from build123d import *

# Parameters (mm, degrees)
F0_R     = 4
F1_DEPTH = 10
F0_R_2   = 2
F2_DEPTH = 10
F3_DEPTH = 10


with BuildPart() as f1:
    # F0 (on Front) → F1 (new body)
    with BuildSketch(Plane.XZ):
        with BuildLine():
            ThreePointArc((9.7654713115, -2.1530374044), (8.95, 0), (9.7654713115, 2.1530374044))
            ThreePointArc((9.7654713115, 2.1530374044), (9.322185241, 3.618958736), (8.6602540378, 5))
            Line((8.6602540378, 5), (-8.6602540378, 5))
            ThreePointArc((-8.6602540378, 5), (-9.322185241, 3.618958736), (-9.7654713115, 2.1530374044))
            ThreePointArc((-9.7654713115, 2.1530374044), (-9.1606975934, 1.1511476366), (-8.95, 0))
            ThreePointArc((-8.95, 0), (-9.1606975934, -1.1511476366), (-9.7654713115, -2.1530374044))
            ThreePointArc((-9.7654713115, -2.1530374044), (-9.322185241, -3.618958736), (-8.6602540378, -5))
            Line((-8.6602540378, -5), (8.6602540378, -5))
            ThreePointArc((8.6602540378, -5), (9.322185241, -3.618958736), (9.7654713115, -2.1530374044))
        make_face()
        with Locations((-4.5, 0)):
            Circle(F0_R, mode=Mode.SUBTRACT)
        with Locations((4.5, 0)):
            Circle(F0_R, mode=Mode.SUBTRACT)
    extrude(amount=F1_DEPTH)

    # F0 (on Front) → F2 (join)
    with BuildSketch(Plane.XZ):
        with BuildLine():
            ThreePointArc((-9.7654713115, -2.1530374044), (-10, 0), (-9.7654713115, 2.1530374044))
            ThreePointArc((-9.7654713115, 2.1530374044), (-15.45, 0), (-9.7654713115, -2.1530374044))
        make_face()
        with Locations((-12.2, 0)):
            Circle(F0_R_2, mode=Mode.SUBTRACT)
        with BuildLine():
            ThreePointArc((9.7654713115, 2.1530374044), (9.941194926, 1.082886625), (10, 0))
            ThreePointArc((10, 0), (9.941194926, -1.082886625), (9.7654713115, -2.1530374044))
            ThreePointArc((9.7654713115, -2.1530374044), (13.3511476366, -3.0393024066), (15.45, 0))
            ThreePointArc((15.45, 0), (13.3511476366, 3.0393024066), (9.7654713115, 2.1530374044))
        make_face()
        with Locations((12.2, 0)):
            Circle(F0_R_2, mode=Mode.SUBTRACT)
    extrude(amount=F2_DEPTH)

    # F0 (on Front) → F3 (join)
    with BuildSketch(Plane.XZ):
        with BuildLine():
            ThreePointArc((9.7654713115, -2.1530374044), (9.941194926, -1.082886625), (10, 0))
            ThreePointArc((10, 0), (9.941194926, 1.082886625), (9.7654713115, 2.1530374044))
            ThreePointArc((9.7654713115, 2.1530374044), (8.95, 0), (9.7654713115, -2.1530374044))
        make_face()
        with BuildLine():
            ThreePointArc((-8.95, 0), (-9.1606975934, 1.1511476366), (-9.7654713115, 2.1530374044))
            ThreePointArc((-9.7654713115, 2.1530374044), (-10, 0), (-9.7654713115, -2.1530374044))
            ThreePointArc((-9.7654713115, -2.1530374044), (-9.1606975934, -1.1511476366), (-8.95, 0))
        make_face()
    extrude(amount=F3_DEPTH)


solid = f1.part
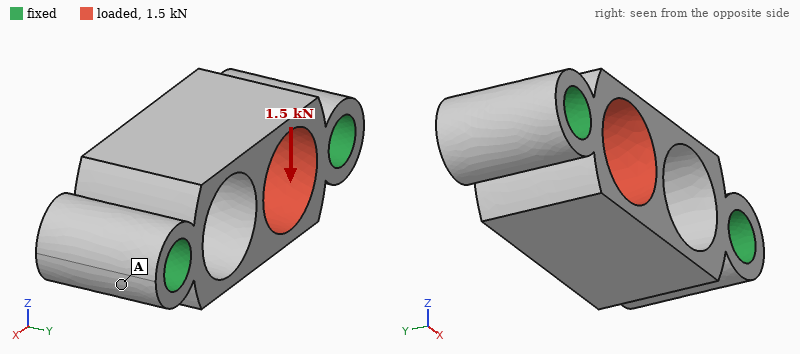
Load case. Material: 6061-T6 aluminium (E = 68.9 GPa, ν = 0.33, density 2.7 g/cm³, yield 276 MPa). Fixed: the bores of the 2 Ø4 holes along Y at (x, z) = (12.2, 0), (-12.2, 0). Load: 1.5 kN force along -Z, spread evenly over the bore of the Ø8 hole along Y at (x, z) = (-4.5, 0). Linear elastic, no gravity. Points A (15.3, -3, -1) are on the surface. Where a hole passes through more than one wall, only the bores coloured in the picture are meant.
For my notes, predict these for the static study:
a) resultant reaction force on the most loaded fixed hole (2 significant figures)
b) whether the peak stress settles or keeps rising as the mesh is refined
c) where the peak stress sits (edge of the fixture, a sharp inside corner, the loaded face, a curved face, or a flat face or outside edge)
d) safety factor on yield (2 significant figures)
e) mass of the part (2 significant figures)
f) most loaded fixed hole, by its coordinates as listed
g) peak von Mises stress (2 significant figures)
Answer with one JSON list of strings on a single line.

["1.1 kN", "settles", "a flat face or outside edge", "1.9", "3.4 g", "(-12.2, 0)", "150 MPa"]
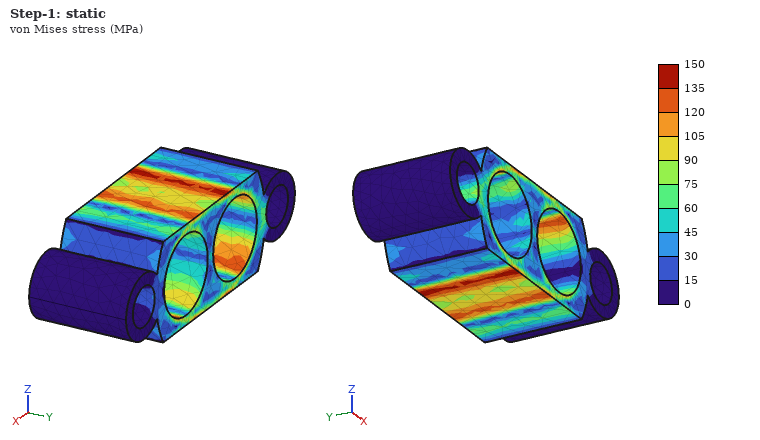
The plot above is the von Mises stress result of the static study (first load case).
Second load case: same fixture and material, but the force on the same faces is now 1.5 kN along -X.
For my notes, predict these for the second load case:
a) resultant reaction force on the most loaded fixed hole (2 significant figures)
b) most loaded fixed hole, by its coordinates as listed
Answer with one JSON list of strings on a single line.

["1.0 kN", "(-12.2, 0)"]
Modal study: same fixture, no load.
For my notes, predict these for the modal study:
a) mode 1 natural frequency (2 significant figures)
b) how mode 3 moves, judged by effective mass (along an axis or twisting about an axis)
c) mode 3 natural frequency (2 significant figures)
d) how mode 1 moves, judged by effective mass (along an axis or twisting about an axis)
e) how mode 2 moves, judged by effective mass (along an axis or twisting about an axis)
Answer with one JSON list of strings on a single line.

["24 kHz", "along Y", "45 kHz", "along Z", "along X"]
